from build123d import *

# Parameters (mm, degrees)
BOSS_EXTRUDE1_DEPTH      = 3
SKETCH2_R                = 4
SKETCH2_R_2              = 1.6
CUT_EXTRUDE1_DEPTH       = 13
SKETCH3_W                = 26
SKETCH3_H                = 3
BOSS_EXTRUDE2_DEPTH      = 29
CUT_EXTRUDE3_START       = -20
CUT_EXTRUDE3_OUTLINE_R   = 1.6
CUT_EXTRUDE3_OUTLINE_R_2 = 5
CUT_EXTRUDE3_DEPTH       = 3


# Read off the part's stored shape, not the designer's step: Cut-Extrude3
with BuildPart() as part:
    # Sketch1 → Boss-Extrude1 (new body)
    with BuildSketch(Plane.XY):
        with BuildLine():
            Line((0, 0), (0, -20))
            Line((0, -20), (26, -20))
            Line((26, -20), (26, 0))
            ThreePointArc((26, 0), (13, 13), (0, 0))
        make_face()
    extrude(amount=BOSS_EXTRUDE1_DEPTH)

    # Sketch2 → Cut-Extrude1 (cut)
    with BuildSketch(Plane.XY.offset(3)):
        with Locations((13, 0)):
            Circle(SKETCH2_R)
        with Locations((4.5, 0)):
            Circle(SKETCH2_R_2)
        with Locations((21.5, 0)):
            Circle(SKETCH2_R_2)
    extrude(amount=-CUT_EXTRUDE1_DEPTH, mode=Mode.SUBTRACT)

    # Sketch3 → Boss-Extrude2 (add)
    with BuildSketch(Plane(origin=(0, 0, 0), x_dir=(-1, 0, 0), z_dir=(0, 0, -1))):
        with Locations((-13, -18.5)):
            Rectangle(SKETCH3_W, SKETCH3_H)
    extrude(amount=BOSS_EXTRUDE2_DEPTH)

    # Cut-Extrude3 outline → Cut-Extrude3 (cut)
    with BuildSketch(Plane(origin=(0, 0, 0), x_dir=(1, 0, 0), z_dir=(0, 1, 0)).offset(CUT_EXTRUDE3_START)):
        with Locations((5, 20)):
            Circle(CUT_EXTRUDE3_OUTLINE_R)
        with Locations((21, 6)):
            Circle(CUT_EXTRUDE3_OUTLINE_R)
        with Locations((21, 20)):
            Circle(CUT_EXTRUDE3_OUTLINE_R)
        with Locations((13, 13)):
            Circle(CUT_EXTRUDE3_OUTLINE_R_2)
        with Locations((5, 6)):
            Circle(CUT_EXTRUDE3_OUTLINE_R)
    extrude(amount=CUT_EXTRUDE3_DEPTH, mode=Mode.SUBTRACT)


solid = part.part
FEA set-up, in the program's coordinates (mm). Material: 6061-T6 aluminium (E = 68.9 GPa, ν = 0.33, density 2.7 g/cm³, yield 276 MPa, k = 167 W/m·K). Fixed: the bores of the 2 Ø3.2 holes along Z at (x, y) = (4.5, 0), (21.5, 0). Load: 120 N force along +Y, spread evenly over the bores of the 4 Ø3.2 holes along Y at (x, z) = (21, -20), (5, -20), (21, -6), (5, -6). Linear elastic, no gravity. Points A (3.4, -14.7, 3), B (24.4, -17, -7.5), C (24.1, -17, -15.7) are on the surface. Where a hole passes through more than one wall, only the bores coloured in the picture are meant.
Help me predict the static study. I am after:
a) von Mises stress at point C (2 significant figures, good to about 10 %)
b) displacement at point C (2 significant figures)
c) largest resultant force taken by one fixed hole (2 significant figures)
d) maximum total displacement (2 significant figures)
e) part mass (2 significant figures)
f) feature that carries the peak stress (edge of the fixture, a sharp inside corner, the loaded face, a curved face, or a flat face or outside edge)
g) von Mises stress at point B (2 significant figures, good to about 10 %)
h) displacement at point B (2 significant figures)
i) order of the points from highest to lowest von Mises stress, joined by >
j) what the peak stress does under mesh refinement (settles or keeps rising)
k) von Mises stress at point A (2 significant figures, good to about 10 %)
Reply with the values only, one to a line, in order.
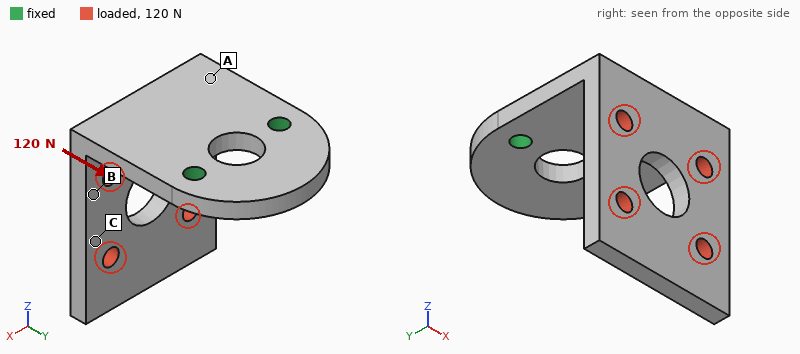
10 MPa
0.19 mm
62 N
0.36 mm
11 g
edge of the fixture
29 MPa
0.10 mm
A > B > C
keeps rising
40 MPa
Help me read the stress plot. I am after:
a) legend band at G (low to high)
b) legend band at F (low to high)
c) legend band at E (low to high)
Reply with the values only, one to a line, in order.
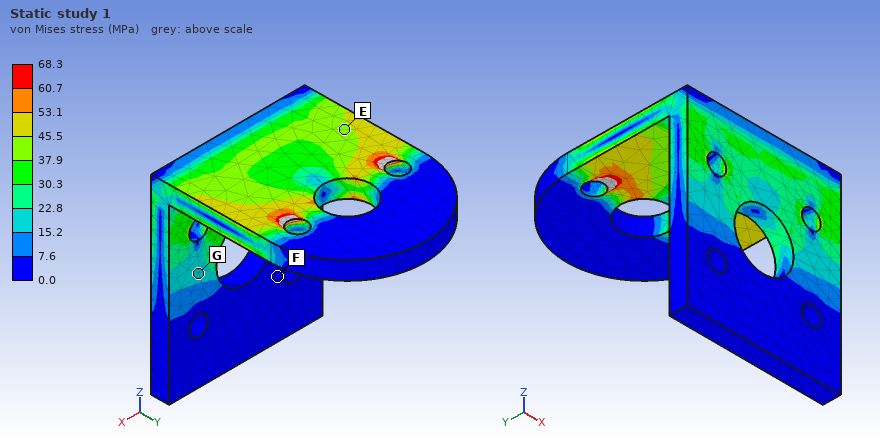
15.2 to 22.8 MPa
0.0 to 7.6 MPa
37.9 to 45.5 MPa
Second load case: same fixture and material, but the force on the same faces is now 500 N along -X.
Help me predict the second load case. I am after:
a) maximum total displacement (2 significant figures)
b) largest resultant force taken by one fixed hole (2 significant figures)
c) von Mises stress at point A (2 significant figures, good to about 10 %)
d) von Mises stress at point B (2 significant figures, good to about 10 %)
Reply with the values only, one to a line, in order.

0.42 mm
640 N
94 MPa
45 MPa
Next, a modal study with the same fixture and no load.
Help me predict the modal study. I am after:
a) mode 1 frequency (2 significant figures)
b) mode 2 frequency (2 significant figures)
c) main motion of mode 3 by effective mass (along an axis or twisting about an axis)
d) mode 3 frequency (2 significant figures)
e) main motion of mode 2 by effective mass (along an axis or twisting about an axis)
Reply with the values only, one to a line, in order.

1300 Hz
2600 Hz
along Z
4000 Hz
along X
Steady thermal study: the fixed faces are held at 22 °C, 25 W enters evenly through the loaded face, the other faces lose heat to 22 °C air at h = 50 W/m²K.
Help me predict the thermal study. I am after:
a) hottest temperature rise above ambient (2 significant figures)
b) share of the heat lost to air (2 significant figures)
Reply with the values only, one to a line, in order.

61 K
21 %
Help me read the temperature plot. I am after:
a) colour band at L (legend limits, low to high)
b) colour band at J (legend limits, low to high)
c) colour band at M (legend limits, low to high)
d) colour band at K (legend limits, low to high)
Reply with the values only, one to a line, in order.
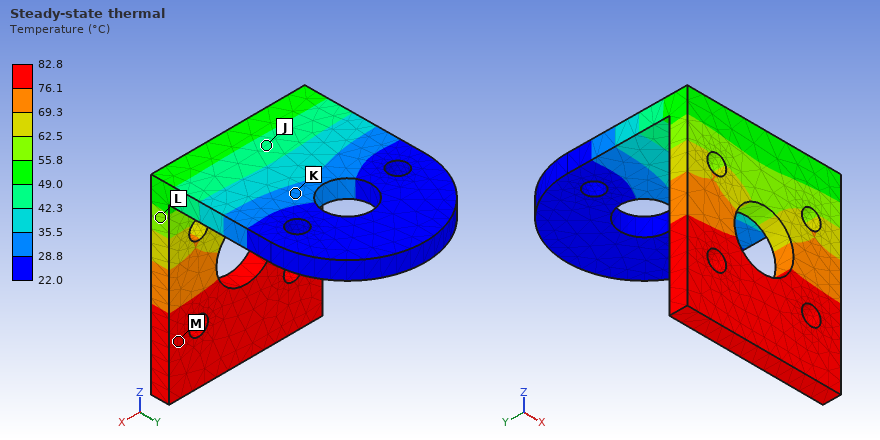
55.8 to 62.5 °C
42.3 to 49.0 °C
76.1 to 82.8 °C
28.8 to 35.5 °C
